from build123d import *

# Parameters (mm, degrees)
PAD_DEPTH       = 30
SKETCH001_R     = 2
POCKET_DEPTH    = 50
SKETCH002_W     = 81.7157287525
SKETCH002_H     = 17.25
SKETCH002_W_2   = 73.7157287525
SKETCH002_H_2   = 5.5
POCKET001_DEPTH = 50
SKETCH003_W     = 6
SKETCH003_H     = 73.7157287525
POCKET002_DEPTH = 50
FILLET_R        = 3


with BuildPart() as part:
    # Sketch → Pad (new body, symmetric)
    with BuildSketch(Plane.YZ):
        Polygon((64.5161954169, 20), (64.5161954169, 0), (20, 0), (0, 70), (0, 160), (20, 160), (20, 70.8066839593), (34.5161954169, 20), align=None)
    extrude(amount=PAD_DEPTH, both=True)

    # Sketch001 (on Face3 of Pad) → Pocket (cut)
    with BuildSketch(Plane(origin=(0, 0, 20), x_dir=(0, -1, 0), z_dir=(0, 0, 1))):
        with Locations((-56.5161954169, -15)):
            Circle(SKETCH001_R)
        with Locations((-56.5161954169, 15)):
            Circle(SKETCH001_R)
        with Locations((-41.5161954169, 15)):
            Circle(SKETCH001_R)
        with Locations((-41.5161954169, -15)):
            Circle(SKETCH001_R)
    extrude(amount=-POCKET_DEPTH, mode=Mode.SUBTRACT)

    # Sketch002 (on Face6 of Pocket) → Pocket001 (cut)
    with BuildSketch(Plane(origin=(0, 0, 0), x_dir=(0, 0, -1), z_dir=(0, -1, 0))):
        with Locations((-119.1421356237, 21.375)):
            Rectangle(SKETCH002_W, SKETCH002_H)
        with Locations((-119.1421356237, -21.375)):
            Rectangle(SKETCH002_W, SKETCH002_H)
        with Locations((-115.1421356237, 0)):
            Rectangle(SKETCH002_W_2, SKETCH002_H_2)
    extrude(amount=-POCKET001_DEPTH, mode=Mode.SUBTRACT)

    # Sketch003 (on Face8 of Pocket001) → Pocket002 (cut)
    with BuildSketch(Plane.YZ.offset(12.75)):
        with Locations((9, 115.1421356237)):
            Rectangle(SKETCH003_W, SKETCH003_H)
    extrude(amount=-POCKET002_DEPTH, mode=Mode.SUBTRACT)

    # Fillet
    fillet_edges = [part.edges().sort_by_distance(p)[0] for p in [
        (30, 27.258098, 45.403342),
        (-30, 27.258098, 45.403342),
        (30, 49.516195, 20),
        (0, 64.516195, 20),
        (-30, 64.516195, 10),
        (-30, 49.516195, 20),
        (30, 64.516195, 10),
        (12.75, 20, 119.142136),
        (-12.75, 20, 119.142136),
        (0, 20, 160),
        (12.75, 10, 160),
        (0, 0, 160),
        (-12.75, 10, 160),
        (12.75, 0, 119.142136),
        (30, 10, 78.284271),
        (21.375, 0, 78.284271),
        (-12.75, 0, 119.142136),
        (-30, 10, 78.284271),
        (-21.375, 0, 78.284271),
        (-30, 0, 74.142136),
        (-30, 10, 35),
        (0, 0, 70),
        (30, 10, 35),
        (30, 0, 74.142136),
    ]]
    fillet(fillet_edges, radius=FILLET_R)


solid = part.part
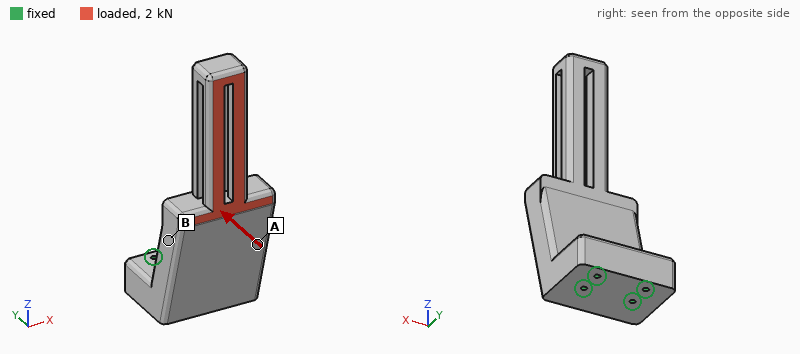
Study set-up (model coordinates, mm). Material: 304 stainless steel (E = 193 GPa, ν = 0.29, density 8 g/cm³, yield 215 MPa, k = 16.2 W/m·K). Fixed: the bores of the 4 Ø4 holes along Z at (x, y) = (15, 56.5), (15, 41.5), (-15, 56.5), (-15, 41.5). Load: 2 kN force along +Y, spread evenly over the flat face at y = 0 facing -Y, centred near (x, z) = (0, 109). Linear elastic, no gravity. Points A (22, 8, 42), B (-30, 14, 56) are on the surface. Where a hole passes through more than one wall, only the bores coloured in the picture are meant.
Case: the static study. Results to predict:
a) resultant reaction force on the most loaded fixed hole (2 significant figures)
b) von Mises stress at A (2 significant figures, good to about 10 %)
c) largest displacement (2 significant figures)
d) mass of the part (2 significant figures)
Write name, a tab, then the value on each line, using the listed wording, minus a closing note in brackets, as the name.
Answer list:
resultant reaction force on the most loaded fixed hole	1.9 kN
von Mises stress at A	34 MPa
largest displacement	0.42 mm
mass of the part	1.2 kg
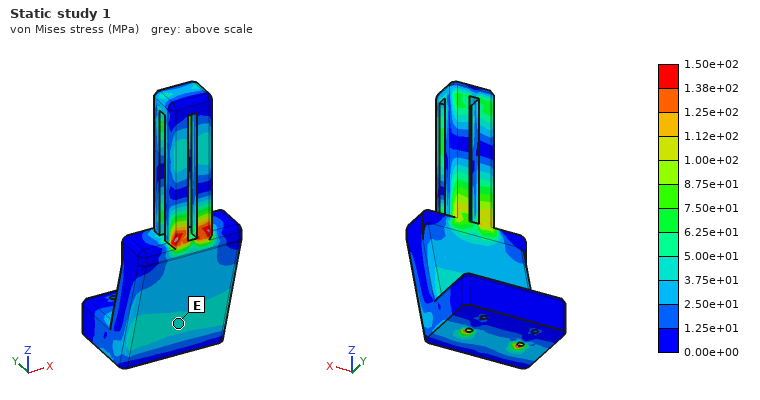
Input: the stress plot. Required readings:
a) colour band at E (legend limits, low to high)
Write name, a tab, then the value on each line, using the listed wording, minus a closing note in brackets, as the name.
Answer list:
colour band at E	3.75e+01 to 5.00e+01 MPa
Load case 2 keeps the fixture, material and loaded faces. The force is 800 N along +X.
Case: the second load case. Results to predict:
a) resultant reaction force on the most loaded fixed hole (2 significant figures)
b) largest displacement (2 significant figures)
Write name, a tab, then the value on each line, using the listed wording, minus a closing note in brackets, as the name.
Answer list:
resultant reaction force on the most loaded fixed hole	1.9 kN
largest displacement	73 µm
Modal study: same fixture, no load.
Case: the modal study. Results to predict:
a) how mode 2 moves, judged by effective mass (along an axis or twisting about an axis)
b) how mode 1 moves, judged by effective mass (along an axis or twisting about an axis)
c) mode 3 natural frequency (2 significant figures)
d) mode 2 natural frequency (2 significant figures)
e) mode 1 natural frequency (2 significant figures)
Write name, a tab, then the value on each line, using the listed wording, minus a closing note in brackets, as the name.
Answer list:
how mode 2 moves, judged by effective mass	along X
how mode 1 moves, judged by effective mass	along Y
mode 3 natural frequency	2400 Hz
mode 2 natural frequency	1300 Hz
mode 1 natural frequency	790 Hz
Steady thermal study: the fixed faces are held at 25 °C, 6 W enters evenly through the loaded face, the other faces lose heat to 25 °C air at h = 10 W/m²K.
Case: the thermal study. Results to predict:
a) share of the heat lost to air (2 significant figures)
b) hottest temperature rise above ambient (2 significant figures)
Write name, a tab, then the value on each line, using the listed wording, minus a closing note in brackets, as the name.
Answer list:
share of the heat lost to air	56 %
hottest temperature rise above ambient	42 K
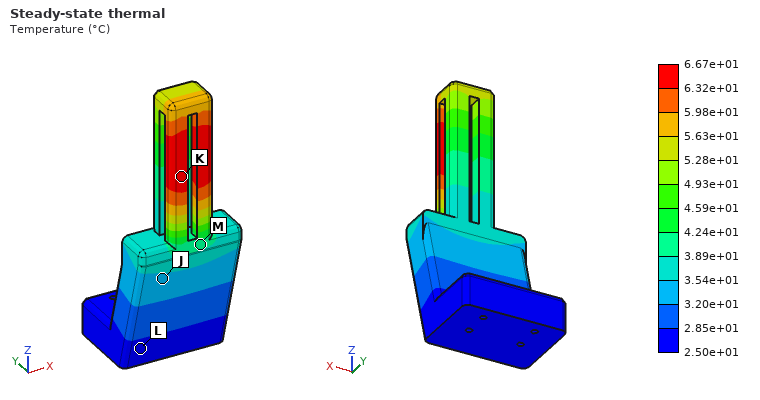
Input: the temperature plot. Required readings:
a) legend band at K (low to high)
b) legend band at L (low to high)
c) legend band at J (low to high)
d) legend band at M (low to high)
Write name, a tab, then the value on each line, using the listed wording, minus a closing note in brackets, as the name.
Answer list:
legend band at K	6.32e+01 to 6.67e+01 °C
legend band at L	2.50e+01 to 2.85e+01 °C
legend band at J	3.20e+01 to 3.54e+01 °C
legend band at M	3.89e+01 to 4.24e+01 °C
